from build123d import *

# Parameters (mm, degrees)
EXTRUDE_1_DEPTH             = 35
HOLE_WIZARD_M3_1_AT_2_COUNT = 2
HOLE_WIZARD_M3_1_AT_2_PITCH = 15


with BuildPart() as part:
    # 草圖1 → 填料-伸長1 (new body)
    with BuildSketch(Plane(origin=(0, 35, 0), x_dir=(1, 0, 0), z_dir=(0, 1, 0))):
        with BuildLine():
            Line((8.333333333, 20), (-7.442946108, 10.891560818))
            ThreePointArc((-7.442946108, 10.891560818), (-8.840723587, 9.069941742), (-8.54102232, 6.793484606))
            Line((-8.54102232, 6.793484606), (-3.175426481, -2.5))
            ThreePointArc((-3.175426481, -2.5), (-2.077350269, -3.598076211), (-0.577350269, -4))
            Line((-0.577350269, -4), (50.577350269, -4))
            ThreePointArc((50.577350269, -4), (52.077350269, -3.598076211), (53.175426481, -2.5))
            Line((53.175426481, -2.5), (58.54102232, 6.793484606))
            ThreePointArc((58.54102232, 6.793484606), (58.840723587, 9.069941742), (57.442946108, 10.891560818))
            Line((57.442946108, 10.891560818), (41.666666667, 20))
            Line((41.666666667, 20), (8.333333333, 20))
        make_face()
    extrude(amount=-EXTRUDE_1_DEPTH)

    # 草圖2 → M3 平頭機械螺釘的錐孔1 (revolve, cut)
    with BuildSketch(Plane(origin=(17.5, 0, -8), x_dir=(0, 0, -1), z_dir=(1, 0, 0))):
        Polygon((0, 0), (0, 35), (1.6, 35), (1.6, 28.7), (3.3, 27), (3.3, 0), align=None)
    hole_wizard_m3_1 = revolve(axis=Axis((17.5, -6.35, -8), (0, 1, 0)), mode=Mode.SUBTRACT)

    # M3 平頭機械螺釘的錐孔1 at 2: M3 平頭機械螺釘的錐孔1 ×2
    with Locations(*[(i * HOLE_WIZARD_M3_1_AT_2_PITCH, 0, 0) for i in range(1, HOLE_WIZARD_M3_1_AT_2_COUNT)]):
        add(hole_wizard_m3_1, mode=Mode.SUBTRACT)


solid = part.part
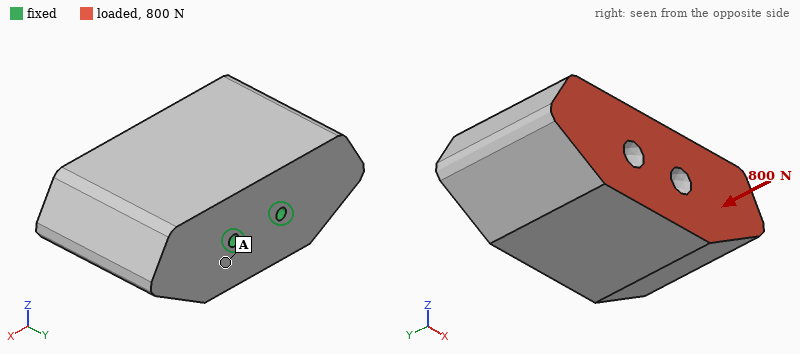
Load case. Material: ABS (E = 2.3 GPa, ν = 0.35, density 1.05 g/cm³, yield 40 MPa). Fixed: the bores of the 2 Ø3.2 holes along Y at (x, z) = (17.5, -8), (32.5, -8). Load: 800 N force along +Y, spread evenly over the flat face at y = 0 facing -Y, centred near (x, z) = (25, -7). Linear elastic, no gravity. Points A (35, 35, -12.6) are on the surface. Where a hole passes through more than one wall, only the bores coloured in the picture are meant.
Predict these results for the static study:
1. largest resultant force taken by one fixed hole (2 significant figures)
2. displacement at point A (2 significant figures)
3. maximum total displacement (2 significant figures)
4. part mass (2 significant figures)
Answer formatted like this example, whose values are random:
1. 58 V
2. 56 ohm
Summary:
1. 400 N
2. 12 µm
3. 55 µm
4. 49 g
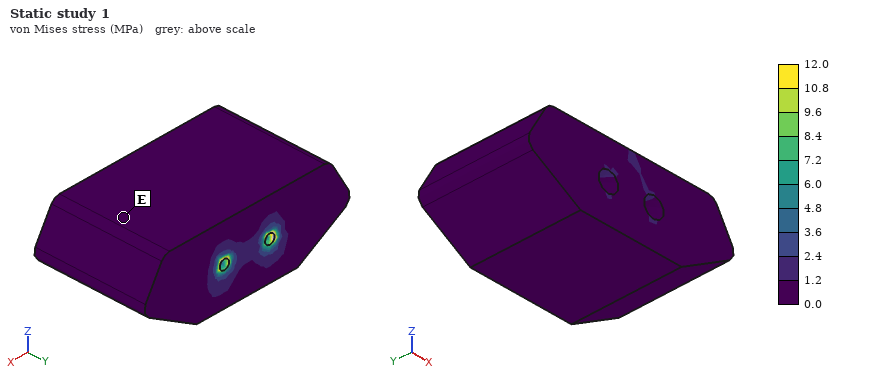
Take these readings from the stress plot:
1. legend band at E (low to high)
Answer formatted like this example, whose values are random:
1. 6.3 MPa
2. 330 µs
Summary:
1. 0.0 to 1.2 MPa
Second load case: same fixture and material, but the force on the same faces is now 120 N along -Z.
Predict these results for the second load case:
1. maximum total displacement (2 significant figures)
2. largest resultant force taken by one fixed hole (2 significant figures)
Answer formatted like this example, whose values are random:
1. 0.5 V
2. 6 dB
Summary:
1. 0.23 mm
2. 60 N
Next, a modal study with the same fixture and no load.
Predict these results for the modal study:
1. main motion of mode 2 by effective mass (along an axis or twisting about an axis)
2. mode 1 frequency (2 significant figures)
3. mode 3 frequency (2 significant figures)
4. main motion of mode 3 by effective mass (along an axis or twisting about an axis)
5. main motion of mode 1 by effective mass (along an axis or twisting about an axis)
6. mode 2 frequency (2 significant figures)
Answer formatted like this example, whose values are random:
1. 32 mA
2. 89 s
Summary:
1. along X
2. 930 Hz
3. 2000 Hz
4. twisting about Y
5. along Z
6. 1500 Hz
